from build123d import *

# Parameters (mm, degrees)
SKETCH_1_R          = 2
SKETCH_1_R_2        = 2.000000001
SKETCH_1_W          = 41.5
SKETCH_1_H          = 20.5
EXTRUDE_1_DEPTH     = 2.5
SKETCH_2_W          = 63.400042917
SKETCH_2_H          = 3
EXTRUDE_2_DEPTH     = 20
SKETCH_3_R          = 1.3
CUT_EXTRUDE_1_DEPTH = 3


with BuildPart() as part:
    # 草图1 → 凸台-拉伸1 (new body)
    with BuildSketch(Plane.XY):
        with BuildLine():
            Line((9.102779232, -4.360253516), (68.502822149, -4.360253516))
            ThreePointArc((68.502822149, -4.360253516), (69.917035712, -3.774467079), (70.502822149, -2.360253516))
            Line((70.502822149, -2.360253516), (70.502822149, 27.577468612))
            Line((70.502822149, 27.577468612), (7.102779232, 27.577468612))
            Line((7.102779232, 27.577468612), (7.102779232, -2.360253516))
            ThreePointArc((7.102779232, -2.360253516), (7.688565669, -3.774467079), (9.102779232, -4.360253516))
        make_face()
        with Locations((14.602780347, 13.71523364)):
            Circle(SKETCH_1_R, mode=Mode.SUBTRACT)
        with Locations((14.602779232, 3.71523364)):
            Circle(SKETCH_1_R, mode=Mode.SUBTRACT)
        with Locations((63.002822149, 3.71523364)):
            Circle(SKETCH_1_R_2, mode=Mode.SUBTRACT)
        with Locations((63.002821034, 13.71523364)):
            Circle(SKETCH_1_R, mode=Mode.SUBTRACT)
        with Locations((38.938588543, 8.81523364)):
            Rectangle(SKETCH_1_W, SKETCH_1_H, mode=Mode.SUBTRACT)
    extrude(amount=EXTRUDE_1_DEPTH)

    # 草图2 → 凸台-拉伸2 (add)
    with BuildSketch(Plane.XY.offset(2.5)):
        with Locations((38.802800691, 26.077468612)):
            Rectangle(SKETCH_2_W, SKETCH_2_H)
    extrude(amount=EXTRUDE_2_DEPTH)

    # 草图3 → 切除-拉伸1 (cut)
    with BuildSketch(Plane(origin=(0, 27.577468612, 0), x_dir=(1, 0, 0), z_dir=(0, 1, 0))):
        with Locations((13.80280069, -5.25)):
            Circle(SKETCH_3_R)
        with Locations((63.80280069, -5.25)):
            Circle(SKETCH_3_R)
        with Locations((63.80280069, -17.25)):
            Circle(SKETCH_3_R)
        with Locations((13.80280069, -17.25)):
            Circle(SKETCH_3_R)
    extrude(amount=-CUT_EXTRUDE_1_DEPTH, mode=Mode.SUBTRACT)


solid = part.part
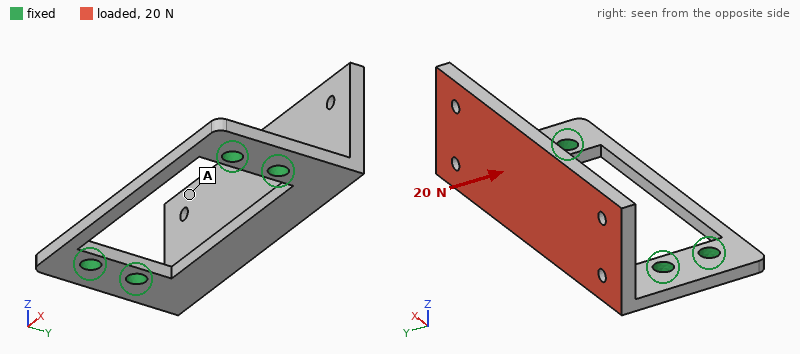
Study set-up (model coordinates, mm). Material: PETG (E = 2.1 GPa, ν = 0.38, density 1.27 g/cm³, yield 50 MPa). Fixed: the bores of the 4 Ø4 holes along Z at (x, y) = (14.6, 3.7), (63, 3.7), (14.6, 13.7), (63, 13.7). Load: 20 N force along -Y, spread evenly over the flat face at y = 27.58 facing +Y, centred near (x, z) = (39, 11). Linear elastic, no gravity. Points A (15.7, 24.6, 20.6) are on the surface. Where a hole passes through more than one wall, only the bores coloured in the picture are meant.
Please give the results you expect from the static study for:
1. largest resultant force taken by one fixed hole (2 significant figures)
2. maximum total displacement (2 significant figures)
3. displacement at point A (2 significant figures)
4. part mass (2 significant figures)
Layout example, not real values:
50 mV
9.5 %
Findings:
11 N
0.83 mm
0.69 mm
8.3 g
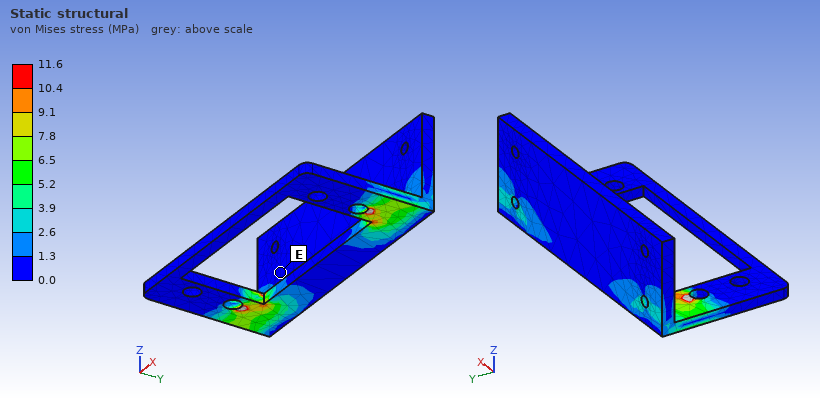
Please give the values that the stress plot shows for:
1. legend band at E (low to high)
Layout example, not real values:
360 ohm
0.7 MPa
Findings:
0.0 to 1.3 MPa
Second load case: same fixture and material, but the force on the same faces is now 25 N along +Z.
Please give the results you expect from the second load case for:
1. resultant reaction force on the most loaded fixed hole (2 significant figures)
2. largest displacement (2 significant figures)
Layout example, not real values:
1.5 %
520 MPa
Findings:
14 N
0.72 mm
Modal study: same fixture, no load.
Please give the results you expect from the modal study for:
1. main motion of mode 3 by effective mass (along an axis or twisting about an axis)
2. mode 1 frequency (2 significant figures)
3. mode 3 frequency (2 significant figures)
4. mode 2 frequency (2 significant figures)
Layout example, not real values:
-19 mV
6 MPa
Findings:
along Z
390 Hz
1400 Hz
940 Hz
